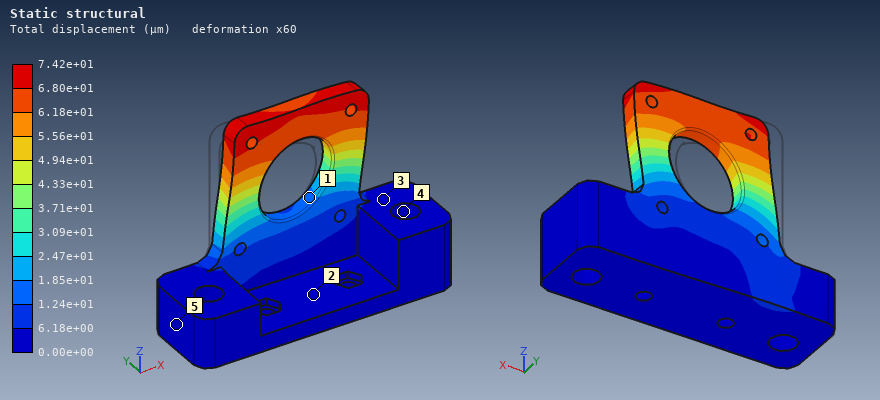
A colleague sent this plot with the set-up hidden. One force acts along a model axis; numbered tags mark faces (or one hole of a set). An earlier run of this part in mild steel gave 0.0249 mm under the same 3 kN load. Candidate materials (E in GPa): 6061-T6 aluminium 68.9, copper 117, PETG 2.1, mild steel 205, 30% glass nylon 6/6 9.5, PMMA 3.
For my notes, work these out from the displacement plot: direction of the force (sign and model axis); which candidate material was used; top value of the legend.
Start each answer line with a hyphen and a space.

- +X
- 6061-T6 aluminium
- 7.42e+01 µm
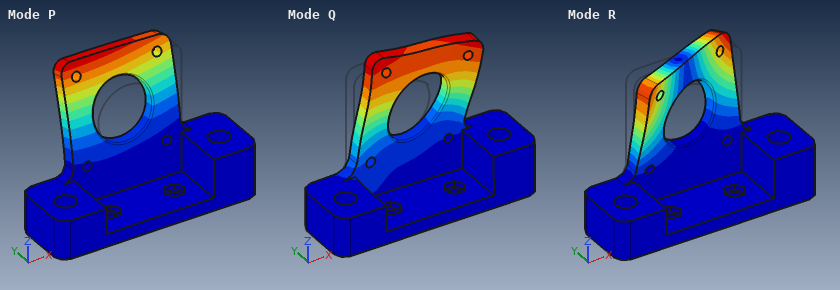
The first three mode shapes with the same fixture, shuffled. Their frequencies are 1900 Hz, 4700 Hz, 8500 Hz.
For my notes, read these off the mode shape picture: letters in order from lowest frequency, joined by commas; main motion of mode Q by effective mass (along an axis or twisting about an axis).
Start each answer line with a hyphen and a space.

- P, R, Q
- along X
